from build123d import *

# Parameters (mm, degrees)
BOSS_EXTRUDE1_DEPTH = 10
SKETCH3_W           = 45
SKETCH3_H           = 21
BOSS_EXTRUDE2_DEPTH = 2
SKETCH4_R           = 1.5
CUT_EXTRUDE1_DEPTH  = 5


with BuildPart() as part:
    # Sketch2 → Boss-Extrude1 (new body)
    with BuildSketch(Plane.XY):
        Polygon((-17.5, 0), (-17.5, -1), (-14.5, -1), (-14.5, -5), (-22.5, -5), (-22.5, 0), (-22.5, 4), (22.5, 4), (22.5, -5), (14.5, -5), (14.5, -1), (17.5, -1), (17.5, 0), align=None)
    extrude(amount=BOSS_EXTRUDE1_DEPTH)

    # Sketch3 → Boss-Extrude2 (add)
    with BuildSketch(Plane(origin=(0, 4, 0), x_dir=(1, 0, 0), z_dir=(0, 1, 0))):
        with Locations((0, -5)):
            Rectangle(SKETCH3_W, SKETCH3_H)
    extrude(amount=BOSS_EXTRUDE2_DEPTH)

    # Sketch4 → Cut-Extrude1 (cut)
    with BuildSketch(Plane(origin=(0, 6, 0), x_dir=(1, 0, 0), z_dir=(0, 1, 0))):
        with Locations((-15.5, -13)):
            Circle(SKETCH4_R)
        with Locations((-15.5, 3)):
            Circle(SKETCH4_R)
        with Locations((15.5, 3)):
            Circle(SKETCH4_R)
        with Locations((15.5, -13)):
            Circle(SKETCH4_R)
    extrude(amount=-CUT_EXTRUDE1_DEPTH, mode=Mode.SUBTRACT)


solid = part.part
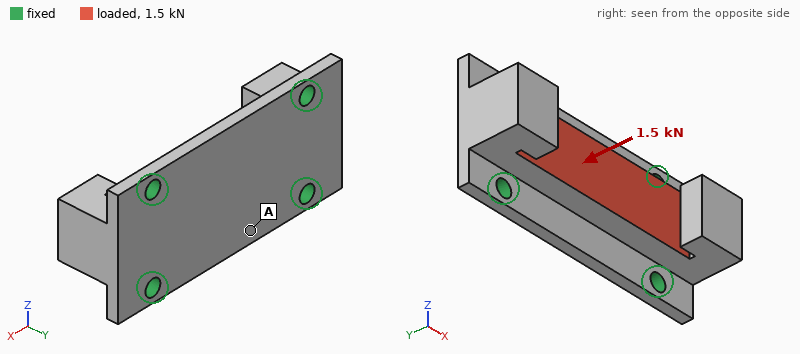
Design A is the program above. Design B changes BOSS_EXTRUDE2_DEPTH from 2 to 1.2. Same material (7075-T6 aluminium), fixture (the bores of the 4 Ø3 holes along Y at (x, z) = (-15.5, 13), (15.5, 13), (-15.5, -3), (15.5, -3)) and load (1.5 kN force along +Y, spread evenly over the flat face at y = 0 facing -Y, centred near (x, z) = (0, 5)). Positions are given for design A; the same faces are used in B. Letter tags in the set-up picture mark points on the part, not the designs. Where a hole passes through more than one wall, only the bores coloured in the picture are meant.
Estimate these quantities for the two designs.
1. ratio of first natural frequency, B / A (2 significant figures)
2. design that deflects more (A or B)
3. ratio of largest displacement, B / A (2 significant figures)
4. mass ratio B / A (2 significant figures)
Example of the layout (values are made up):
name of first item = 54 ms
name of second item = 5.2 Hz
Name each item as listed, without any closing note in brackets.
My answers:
ratio of first natural frequency, B / A = 0.82
design that deflects more = B
ratio of largest displacement, B / A = 1.9
mass ratio B / A = 0.83
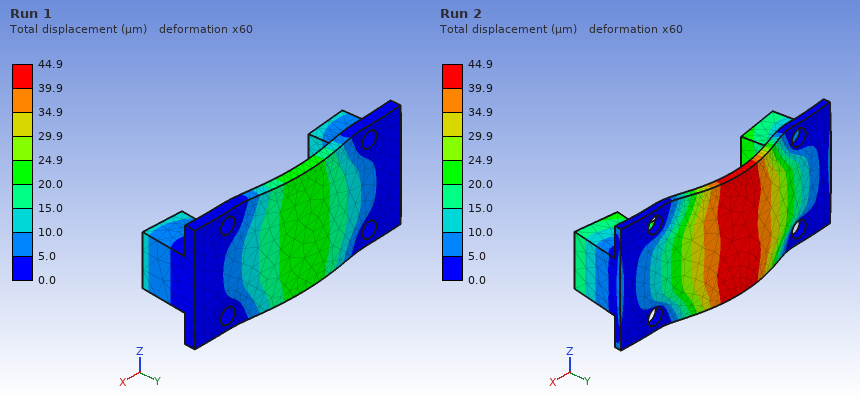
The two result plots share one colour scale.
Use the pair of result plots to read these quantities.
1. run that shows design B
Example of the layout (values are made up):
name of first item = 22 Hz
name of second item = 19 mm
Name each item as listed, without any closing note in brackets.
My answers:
run that shows design B = Run 2
